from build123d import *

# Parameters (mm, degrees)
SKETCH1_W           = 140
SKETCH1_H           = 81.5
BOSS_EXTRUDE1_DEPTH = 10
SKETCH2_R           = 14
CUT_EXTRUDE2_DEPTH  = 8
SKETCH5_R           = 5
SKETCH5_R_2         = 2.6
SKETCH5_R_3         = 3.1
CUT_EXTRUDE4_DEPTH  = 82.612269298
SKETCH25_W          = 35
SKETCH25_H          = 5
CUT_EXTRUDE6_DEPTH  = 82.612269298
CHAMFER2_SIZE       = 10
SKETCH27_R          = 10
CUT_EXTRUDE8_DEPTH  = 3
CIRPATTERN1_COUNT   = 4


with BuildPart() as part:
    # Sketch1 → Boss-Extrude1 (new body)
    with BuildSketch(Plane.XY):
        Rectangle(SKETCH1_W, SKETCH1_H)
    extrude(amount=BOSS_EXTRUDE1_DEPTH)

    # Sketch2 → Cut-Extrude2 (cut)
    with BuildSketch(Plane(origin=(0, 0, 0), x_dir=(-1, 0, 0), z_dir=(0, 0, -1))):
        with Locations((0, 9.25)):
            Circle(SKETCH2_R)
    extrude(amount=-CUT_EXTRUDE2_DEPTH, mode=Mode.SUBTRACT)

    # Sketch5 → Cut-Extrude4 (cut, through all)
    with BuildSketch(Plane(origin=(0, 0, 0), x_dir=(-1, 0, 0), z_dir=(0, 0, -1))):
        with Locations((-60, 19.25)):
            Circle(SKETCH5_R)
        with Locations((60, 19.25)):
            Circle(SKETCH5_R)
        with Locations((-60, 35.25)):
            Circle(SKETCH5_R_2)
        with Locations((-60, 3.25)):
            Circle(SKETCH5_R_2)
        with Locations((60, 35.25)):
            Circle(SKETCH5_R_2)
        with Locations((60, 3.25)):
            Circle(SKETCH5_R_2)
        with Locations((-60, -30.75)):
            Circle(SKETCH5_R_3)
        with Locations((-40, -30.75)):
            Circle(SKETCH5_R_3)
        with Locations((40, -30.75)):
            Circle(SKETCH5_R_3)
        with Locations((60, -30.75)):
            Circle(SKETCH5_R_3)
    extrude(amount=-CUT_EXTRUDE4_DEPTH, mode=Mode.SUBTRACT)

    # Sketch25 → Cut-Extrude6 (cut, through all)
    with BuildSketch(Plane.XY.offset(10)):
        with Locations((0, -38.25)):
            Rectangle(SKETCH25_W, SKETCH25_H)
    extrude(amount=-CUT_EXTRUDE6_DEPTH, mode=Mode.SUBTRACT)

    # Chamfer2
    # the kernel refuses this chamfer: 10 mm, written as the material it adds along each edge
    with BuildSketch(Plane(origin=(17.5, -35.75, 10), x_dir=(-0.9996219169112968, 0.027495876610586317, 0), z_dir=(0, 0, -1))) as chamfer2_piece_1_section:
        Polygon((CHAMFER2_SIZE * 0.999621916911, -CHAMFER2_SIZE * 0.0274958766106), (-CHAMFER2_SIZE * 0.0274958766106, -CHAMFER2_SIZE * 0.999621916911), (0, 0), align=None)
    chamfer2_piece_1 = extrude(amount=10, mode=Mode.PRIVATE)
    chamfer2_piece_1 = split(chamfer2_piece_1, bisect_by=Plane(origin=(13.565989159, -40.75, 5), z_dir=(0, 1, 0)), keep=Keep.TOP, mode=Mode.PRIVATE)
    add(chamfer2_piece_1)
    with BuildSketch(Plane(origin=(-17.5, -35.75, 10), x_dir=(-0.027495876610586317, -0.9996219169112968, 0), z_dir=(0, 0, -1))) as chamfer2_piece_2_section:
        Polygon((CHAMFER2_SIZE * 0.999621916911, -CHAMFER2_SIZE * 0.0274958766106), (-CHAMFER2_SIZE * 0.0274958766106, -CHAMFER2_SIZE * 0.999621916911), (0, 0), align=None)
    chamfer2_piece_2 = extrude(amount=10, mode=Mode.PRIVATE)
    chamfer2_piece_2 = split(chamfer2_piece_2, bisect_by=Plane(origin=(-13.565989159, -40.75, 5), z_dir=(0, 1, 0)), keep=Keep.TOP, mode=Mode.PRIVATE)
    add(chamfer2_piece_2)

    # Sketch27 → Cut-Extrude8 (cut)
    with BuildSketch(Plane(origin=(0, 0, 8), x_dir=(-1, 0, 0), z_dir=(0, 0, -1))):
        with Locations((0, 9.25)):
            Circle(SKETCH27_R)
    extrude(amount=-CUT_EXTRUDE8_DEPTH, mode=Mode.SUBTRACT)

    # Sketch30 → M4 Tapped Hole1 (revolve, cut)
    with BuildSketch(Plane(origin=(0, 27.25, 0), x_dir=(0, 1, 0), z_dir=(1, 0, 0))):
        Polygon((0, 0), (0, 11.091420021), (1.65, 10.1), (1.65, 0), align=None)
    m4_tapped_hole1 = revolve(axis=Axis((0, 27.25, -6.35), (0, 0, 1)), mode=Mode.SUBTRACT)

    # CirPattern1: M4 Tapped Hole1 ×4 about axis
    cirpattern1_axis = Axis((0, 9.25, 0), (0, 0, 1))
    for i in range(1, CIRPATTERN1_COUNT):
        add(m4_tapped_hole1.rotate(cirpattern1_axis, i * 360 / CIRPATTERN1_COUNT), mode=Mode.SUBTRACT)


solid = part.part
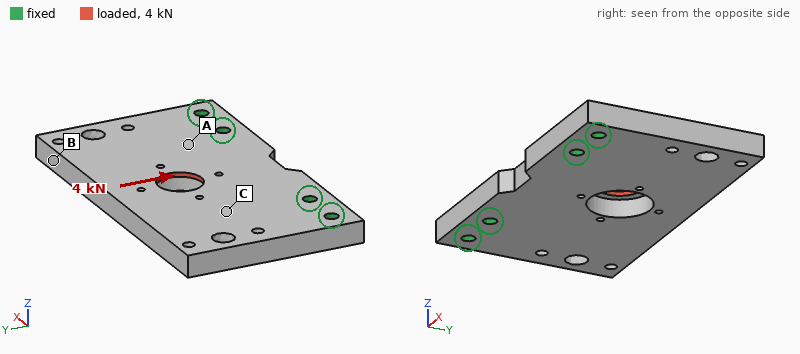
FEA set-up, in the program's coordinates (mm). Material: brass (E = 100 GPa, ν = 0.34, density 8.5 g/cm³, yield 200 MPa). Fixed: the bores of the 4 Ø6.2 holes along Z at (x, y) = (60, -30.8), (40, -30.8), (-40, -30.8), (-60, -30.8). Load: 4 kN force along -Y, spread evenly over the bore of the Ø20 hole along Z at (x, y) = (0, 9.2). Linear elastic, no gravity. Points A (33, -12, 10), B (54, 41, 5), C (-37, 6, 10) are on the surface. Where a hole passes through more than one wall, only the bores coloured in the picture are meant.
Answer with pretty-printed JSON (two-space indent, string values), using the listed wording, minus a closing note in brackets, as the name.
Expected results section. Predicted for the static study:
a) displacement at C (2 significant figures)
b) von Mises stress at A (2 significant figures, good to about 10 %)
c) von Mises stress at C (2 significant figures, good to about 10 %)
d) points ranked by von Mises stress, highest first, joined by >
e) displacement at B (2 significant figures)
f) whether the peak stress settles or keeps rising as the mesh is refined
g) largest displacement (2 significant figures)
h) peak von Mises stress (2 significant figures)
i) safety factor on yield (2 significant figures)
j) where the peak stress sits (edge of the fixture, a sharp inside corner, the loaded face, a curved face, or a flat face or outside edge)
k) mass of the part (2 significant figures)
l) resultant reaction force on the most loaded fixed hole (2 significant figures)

{
  "displacement at C": "13 µm",
  "von Mises stress at A": "12 MPa",
  "von Mises stress at C": "8.5 MPa",
  "points ranked by von Mises stress, highest first, joined by >": "A > C > B",
  "displacement at B": "30 µm",
  "whether the peak stress settles or keeps rising as the mesh is refined": "settles",
  "largest displacement": "41 µm",
  "peak von Mises stress": "61 MPa",
  "safety factor on yield": "3.3",
  "where the peak stress sits": "the loaded face",
  "mass of the part": "880 g",
  "resultant reaction force on the most loaded fixed hole": "1.7 kN"
}
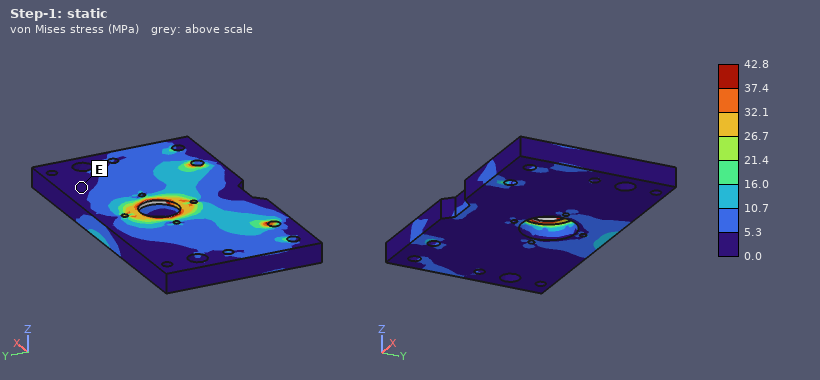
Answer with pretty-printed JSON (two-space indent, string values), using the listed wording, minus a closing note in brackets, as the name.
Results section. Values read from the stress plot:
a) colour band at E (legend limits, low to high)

{
  "colour band at E": "0.0 to 5.3 MPa"
}
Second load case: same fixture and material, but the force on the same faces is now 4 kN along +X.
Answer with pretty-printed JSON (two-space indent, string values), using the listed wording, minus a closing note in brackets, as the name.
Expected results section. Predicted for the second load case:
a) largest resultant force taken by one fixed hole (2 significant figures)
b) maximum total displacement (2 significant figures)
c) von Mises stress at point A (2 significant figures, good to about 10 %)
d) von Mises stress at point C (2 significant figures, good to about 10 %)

{
  "largest resultant force taken by one fixed hole": "1.4 kN",
  "maximum total displacement": "14 µm",
  "von Mises stress at point A": "7.3 MPa",
  "von Mises stress at point C": "7.4 MPa"
}
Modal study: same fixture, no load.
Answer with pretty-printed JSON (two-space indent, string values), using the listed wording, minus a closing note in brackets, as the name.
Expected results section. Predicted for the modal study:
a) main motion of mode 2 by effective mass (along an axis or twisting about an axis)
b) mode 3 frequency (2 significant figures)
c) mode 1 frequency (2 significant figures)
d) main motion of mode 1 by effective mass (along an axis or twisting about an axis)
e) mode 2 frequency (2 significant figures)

{
  "main motion of mode 2 by effective mass": "twisting about Y",
  "mode 3 frequency": "2900 Hz",
  "mode 1 frequency": "970 Hz",
  "main motion of mode 1 by effective mass": "along Z",
  "mode 2 frequency": "1600 Hz"
}
